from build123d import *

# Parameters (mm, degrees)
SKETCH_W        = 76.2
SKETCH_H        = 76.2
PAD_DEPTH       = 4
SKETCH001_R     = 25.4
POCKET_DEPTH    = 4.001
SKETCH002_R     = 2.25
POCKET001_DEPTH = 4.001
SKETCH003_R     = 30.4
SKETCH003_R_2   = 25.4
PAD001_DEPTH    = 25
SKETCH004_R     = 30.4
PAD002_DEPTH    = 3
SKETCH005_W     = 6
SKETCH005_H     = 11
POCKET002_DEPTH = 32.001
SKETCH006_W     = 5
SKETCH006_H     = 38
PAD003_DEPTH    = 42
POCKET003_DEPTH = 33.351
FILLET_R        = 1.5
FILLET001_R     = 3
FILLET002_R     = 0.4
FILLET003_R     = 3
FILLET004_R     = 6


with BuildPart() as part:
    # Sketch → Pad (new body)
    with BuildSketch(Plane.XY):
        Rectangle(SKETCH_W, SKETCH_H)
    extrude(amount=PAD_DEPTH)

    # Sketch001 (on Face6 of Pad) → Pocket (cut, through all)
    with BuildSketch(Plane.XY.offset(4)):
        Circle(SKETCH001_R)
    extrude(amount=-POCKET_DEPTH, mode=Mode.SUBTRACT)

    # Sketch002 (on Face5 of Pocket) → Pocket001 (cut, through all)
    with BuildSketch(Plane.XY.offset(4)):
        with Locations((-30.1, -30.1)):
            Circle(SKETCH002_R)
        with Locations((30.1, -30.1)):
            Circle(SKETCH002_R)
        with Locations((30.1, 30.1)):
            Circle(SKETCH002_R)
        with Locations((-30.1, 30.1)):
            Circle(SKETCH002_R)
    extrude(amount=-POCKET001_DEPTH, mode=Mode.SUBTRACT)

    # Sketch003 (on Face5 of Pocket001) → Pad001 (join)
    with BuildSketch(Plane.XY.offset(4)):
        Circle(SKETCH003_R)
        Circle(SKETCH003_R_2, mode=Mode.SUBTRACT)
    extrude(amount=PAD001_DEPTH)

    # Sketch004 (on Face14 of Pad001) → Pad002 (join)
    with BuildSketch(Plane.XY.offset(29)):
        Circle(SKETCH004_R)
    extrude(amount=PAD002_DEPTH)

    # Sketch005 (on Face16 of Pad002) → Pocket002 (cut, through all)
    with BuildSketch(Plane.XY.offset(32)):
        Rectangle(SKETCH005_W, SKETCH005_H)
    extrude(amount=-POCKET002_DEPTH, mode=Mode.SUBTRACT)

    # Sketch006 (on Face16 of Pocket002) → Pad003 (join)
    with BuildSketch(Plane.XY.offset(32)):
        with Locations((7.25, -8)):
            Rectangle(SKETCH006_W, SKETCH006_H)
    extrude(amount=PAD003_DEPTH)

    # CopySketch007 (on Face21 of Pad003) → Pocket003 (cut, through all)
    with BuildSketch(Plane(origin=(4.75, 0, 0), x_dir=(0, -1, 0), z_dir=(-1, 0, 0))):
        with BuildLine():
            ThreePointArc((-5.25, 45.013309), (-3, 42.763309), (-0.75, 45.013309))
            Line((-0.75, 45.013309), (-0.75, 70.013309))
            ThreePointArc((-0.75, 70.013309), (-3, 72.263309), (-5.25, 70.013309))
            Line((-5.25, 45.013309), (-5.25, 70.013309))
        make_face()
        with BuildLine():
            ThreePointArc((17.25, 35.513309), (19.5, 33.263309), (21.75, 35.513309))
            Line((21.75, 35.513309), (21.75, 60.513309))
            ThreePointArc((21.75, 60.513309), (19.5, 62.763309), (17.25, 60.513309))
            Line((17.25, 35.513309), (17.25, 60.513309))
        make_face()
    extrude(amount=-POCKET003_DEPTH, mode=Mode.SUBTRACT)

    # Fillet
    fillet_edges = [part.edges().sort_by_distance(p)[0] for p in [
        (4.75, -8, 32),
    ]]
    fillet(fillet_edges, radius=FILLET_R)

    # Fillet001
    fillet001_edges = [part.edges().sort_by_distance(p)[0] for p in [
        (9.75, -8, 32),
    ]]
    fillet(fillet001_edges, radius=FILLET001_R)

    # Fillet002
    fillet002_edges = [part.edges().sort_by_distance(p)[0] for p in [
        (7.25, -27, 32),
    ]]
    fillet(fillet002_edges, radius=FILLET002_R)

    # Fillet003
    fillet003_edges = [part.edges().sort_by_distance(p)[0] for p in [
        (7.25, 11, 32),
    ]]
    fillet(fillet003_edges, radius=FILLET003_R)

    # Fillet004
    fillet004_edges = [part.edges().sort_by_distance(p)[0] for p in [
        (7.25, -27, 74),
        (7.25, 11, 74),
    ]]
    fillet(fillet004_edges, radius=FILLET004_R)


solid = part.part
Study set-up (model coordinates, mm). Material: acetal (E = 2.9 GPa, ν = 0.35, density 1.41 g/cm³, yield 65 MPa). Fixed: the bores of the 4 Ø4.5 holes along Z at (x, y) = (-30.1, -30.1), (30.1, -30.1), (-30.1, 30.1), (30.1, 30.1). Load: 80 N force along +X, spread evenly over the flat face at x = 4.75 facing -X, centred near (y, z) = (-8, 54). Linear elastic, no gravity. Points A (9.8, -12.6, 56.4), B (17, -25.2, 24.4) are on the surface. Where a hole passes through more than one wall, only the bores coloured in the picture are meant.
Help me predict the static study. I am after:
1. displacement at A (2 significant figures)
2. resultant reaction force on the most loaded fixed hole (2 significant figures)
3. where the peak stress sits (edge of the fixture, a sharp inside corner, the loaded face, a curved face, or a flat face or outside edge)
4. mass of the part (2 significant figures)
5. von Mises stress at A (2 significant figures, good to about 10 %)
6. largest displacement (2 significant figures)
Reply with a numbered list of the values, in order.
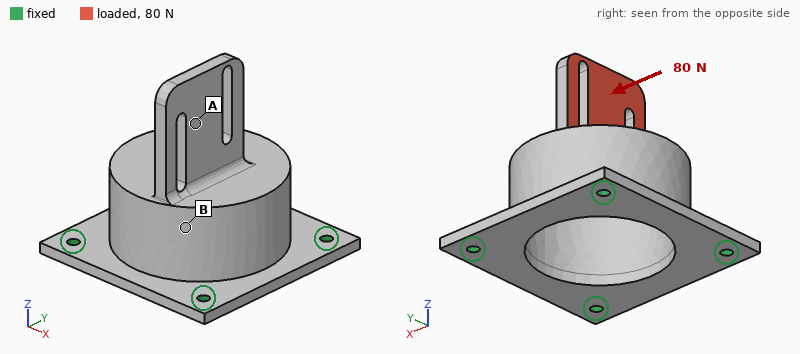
1. 0.68 mm
2. 47 N
3. the loaded face
4. 73 g
5. 2.8 MPa
6. 1.3 mm
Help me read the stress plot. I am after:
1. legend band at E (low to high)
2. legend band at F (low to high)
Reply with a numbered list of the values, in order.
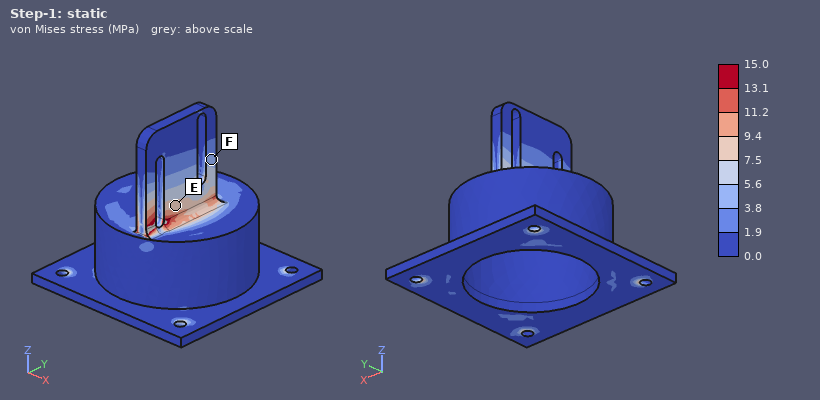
1. 7.5 to 9.4 MPa
2. 3.8 to 5.6 MPa
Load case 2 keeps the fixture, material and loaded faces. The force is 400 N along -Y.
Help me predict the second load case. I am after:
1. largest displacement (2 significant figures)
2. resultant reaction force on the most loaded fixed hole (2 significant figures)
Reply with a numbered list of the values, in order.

1. 1.3 mm
2. 230 N
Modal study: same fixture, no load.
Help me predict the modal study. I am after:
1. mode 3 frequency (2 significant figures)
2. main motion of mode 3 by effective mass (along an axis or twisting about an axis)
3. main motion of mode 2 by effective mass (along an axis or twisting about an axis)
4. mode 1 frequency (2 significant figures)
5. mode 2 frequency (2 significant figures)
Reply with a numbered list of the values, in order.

1. 1200 Hz
2. along Z
3. along Y
4. 510 Hz
5. 910 Hz
